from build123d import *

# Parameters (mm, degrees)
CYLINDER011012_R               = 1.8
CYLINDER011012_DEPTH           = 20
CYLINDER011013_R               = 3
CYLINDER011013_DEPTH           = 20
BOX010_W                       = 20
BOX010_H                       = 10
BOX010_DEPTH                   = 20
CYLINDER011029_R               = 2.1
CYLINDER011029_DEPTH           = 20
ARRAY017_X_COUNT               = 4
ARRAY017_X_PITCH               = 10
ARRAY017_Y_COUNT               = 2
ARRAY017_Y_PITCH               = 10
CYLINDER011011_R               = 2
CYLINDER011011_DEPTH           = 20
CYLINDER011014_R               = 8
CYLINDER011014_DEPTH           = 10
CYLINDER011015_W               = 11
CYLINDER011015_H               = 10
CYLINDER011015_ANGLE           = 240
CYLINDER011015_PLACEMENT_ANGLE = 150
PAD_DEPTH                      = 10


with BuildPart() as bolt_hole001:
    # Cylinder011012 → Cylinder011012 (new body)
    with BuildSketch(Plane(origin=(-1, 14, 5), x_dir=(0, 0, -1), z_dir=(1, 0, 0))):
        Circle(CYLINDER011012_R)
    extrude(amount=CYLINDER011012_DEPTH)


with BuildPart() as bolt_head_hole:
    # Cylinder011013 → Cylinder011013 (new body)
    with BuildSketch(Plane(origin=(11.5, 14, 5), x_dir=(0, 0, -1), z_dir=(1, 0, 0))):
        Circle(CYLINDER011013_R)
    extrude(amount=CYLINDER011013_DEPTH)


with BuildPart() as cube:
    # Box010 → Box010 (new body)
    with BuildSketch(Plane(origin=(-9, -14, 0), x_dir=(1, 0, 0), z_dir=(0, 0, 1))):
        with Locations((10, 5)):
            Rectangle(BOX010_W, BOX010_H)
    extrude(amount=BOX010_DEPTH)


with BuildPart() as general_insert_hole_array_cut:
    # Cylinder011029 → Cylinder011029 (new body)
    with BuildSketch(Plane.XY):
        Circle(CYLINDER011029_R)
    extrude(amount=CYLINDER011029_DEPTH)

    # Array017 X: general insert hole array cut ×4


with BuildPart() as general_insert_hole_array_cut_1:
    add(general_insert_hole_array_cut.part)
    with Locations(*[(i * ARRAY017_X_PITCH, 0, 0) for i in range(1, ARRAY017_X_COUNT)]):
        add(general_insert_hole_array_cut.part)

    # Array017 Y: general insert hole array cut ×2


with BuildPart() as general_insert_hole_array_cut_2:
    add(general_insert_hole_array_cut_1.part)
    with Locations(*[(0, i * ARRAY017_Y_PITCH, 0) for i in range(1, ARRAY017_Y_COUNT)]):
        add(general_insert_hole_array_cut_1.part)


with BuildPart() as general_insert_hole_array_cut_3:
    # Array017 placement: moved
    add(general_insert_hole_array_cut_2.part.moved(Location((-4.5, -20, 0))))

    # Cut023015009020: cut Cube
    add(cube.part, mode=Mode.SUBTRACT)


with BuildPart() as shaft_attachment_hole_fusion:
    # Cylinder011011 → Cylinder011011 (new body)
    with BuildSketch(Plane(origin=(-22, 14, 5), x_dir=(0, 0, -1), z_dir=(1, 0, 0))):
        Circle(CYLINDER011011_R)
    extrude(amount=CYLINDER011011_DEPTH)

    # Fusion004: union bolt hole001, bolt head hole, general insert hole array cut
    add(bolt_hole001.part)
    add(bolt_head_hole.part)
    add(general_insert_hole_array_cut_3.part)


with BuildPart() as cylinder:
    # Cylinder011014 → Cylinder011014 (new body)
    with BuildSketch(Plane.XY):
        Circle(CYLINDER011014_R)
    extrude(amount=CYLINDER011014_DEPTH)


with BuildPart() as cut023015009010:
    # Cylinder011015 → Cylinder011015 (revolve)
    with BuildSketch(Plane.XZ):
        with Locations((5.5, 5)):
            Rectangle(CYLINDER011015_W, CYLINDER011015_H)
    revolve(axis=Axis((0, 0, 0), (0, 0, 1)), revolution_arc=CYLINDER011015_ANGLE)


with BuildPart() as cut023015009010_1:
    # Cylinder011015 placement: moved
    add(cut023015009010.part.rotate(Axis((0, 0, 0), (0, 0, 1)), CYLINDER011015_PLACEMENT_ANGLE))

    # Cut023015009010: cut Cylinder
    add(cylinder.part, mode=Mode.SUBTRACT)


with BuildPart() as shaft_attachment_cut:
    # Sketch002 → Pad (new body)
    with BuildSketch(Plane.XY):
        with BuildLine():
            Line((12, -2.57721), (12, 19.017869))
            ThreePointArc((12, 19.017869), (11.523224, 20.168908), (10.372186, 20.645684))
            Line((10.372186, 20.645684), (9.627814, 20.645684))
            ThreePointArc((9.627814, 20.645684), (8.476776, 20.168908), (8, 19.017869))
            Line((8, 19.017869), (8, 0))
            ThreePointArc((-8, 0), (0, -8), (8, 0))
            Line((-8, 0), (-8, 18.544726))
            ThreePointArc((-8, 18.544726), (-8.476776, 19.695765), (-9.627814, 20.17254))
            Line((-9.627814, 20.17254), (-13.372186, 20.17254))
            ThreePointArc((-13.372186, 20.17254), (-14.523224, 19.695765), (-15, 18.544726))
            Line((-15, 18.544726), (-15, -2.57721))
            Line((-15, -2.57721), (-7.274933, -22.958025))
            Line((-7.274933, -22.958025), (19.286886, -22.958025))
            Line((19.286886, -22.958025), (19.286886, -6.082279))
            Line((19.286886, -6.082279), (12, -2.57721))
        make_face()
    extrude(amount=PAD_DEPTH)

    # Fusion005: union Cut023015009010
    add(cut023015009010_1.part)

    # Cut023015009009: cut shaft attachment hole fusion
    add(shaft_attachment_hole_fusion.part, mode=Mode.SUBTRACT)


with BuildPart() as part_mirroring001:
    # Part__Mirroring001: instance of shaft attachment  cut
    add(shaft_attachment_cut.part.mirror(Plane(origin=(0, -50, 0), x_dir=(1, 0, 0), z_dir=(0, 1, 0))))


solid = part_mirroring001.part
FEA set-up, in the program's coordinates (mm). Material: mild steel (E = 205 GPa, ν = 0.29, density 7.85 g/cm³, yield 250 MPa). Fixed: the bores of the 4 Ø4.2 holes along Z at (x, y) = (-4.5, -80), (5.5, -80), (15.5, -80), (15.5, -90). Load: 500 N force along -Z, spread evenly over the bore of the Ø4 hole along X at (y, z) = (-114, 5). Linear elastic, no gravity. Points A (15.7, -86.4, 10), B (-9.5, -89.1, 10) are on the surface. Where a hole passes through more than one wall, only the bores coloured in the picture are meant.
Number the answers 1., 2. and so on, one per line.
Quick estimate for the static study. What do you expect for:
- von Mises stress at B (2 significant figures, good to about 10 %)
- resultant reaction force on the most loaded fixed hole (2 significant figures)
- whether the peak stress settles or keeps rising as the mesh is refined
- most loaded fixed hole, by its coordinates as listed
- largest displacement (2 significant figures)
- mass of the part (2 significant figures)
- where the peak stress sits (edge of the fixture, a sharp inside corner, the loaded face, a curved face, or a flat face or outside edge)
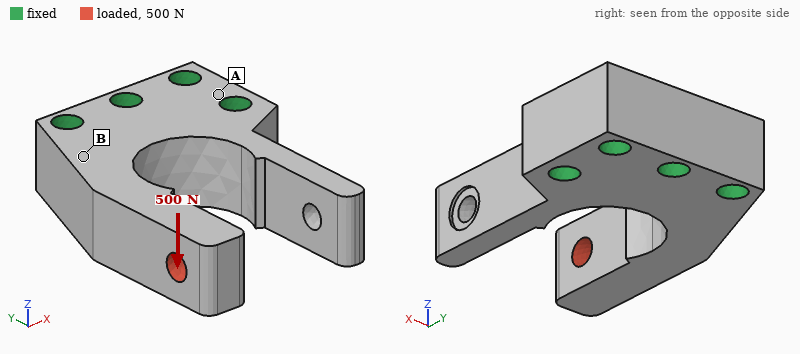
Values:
1. 88 MPa
2. 320 N
3. keeps rising
4. (-4.5, -80)
5. 58 µm
6. 57 g
7. edge of the fixture
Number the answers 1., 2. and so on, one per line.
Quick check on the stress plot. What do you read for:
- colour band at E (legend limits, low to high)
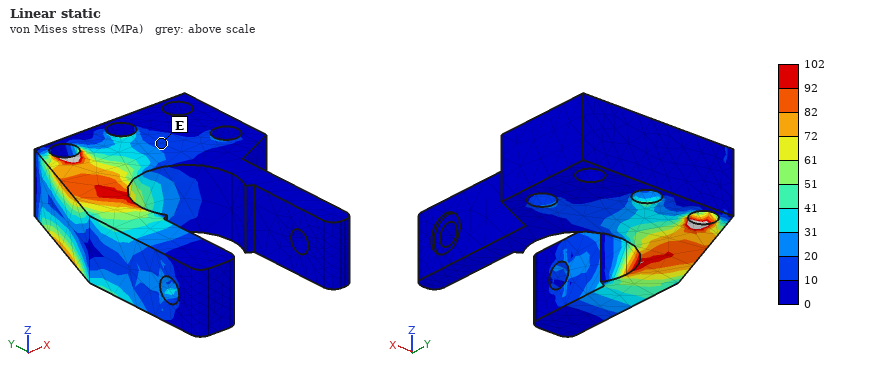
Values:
1. 10 to 20 MPa
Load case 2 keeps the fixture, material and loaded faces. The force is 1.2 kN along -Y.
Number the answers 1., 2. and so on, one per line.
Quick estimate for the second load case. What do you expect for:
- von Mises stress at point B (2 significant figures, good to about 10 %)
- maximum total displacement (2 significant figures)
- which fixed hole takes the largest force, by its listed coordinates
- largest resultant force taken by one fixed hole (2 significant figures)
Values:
1. 29 MPa
2. 17 µm
3. (-4.5, -80)
4. 1.6 kN
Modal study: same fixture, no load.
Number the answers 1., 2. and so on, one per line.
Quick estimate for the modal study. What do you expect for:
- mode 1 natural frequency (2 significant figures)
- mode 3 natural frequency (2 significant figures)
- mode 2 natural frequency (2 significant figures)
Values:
1. 5800 Hz
2. 5900 Hz
3. 5900 Hz
